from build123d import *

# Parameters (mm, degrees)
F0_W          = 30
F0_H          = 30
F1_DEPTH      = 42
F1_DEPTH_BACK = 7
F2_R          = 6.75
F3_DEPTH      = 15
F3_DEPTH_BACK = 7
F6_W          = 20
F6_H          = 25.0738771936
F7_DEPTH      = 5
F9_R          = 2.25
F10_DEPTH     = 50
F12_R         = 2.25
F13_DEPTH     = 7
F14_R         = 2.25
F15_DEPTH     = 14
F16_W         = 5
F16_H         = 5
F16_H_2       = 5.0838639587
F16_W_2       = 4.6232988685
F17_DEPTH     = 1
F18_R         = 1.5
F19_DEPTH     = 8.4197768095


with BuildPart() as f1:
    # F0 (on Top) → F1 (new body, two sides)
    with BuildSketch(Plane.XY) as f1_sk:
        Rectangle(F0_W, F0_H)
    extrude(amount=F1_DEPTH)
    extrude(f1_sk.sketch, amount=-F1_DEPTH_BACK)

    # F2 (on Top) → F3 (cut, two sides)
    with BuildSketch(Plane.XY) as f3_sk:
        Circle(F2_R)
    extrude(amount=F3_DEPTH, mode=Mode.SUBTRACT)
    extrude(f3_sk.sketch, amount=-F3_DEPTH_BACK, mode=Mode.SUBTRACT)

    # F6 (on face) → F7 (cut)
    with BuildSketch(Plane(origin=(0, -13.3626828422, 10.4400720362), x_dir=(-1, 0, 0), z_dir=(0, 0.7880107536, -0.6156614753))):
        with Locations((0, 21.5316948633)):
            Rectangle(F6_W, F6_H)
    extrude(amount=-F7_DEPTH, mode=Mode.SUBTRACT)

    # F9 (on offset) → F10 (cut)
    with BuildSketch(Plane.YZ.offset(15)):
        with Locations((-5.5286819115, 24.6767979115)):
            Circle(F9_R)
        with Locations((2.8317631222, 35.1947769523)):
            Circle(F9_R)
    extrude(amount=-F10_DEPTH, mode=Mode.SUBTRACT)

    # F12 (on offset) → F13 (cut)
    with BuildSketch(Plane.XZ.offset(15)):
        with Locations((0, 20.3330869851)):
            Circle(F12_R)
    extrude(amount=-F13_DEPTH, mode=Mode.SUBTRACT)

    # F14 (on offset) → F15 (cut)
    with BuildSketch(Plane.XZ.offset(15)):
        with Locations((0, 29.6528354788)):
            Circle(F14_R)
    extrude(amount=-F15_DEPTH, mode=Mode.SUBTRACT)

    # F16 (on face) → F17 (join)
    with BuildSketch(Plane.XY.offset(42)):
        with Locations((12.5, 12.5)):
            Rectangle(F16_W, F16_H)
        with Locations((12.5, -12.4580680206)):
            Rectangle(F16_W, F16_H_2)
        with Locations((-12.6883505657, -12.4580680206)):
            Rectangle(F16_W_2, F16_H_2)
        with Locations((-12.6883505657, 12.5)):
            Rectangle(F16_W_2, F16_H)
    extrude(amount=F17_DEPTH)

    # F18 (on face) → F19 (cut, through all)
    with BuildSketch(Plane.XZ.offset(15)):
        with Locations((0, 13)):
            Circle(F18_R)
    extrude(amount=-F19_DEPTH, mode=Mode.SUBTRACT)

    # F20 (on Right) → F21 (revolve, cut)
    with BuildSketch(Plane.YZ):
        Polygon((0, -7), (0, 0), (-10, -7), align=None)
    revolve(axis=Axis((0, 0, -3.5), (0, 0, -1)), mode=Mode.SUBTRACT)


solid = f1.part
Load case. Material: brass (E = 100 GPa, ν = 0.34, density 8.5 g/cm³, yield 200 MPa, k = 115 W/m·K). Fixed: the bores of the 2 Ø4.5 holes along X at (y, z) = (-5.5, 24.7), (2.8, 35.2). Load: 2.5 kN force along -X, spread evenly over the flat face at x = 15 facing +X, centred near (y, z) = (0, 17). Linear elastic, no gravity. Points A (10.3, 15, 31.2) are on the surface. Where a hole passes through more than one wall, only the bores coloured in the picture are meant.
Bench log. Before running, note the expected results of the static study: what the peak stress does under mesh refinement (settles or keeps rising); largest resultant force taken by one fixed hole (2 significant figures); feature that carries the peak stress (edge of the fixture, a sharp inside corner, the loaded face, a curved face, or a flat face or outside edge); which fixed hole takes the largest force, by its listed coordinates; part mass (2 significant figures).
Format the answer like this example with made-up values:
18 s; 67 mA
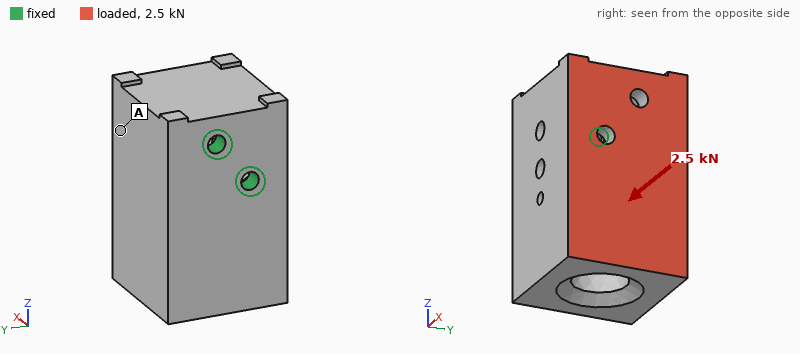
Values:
keeps rising; 2.5 kN; edge of the fixture; (-5.5, 24.7); 320 g
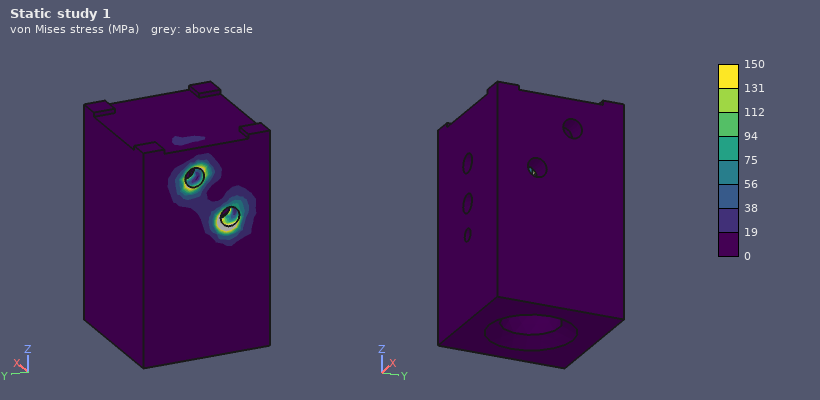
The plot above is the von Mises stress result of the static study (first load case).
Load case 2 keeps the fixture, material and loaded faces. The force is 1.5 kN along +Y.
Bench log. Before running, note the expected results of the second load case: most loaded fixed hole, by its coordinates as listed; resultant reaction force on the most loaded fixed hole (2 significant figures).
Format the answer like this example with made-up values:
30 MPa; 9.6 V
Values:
(-5.5, 24.7); 2.3 kN
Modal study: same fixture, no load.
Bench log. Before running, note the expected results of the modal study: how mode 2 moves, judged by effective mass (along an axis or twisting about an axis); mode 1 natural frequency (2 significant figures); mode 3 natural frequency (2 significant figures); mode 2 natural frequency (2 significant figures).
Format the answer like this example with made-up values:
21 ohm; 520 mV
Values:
along Y; 1800 Hz; 5100 Hz; 3500 Hz
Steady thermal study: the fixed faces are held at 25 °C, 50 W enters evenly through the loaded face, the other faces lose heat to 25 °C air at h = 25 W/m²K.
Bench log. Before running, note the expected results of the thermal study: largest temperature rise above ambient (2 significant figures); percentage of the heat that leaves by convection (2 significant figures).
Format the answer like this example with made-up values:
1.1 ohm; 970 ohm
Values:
23 K; 6.2 %
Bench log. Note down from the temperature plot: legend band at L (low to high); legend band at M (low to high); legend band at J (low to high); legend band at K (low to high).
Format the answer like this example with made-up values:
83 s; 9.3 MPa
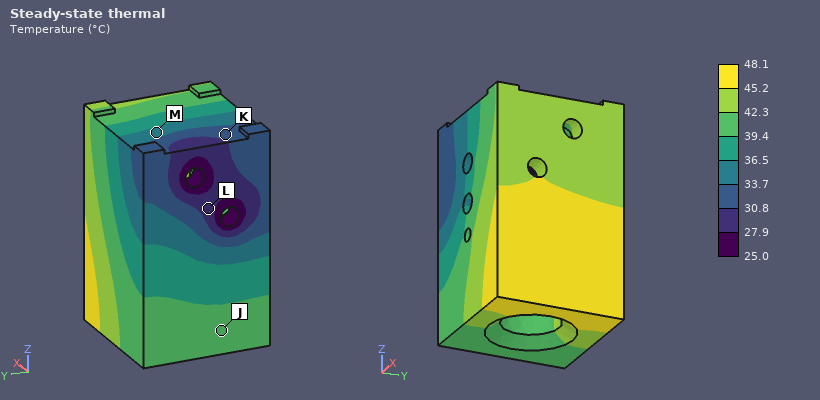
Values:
27.9 to 30.8 °C; 33.7 to 36.5 °C; 39.4 to 42.3 °C; 30.8 to 33.7 °C
